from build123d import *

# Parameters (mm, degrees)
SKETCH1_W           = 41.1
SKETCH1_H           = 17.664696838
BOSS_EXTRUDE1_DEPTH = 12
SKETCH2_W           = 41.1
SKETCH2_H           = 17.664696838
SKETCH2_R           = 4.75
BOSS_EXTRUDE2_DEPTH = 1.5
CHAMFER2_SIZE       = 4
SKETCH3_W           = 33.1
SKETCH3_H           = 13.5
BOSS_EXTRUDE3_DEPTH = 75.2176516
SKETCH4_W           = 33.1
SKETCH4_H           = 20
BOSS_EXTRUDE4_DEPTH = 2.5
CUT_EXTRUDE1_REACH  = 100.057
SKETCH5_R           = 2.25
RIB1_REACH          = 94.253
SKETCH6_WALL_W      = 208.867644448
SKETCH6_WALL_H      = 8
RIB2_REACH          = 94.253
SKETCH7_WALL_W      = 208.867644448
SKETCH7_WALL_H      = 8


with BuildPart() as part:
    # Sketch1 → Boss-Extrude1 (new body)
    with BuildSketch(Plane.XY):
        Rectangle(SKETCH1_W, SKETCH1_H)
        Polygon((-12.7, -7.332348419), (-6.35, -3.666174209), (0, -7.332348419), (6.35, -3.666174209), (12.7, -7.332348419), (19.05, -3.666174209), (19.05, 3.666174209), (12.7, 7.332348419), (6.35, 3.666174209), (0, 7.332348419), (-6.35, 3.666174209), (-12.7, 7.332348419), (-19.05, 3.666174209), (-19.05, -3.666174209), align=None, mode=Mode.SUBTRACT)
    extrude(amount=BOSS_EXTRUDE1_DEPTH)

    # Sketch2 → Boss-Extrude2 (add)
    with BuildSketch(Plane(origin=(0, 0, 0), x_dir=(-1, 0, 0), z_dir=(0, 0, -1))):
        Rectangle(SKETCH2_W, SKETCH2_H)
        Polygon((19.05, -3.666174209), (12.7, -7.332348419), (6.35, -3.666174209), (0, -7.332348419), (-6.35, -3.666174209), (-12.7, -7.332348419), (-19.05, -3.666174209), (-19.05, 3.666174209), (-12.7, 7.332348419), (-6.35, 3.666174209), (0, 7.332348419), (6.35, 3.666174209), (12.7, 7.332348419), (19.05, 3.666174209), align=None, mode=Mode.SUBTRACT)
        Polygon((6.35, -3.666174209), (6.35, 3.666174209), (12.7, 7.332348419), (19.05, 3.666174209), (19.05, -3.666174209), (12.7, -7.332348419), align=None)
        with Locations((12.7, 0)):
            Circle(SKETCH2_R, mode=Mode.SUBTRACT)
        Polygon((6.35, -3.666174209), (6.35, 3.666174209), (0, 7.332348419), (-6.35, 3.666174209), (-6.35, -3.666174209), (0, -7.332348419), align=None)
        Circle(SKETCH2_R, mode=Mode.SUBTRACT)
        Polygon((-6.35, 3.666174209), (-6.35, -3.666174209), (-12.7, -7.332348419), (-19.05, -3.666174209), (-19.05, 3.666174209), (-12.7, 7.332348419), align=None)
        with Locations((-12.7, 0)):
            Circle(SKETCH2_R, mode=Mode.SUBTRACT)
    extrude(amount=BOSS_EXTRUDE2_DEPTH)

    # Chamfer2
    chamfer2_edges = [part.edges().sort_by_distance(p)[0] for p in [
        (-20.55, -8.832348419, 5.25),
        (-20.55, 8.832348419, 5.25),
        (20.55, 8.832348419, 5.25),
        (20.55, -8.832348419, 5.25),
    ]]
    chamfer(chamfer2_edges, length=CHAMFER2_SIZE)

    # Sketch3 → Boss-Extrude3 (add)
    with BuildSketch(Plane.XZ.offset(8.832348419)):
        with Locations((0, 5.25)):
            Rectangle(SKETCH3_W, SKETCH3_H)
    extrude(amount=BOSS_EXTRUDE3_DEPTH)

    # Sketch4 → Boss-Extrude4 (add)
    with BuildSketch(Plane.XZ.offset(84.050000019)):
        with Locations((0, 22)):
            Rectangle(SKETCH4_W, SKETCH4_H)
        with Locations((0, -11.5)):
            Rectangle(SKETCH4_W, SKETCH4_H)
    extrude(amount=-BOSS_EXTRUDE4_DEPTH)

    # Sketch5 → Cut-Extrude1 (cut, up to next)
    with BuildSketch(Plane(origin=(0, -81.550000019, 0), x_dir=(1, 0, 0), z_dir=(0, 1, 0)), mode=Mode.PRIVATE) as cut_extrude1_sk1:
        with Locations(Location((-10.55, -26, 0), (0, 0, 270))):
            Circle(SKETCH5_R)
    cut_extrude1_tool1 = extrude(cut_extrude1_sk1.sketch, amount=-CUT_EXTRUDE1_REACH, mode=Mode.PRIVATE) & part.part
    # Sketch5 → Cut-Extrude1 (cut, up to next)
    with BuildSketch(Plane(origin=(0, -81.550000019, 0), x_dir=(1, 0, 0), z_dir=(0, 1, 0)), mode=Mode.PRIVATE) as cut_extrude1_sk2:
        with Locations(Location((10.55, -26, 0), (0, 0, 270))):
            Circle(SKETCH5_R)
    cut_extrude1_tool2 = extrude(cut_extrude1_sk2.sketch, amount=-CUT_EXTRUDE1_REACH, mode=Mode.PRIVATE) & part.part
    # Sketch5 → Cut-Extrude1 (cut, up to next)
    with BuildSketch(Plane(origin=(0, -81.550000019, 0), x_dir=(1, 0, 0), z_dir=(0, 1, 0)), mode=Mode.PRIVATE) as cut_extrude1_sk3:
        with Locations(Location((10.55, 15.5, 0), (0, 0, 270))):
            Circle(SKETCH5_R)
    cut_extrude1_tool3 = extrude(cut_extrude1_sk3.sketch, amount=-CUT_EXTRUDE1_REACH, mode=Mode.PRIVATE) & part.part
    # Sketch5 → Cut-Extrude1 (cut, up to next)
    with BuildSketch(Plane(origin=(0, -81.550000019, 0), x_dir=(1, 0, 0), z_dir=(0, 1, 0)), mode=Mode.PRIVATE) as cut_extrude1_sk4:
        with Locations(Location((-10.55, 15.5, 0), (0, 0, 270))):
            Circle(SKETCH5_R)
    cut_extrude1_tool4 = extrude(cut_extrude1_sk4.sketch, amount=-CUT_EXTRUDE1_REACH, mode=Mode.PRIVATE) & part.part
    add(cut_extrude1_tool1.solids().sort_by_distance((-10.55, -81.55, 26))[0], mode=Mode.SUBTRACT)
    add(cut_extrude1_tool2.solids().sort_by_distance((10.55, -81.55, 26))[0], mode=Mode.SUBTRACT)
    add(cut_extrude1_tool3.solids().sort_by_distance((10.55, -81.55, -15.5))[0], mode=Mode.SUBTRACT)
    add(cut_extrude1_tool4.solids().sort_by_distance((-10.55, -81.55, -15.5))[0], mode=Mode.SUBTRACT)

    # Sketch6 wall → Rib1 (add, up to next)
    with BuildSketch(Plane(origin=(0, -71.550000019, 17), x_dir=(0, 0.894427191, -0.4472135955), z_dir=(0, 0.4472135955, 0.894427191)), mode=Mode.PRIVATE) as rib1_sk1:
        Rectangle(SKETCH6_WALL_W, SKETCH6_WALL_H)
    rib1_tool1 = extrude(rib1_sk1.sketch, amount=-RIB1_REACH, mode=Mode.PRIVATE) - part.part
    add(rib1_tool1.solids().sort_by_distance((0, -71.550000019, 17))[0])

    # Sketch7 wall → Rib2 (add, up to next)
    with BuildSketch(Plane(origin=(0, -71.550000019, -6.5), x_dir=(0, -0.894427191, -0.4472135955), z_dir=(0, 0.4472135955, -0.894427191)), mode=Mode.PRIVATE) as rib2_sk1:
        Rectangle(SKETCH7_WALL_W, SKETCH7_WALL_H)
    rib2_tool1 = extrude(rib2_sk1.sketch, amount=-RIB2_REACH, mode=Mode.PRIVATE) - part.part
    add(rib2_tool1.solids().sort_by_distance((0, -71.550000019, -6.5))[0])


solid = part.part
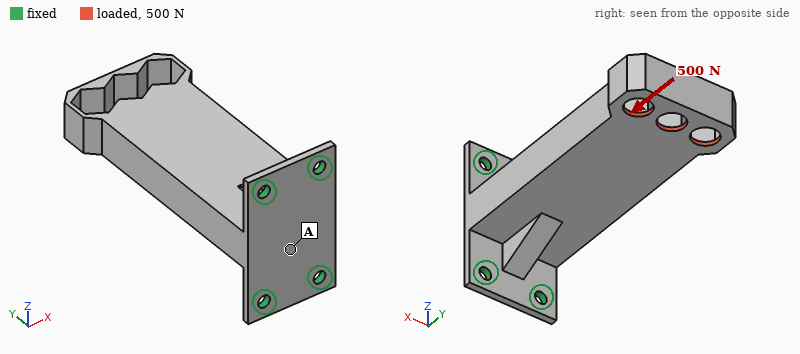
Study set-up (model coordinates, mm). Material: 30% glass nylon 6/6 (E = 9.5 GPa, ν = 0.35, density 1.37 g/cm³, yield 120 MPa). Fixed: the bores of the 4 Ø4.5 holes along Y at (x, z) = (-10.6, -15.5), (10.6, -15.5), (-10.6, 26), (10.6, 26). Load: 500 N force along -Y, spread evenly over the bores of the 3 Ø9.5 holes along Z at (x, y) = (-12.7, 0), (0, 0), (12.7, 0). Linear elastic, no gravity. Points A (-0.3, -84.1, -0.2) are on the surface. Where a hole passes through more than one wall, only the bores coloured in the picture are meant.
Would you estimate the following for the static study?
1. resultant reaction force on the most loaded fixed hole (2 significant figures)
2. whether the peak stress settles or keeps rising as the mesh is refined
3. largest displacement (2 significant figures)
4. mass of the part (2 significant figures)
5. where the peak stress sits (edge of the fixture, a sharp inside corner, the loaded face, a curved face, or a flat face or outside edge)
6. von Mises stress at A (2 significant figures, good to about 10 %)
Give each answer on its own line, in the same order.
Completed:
190 N
keeps rising
0.30 mm
58 g
edge of the fixture
4.8 MPa
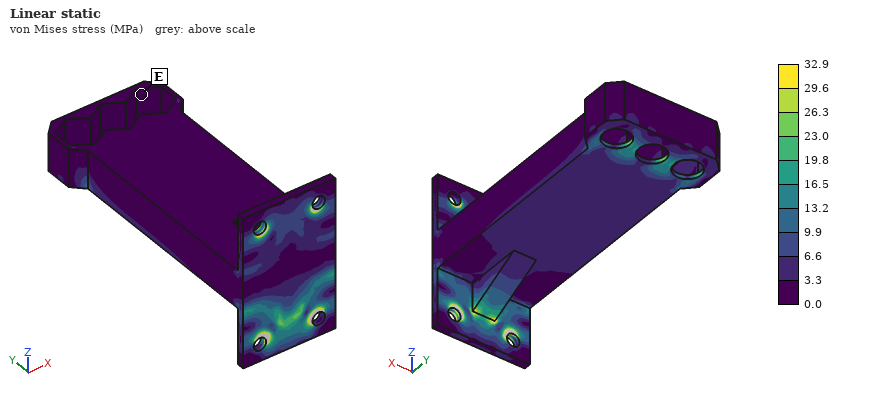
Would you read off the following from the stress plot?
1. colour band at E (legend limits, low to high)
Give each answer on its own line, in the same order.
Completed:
0.0 to 3.3 MPa
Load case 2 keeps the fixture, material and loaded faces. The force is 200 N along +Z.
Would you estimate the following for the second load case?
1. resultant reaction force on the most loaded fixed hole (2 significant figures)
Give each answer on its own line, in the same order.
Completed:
250 N
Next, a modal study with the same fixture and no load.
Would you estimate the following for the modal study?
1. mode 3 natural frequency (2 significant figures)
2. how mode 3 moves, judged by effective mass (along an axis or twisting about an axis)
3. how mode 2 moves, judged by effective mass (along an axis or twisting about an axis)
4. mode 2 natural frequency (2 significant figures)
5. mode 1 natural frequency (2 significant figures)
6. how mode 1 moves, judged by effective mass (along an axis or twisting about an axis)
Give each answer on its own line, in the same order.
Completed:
1900 Hz
along Y
along Z
590 Hz
330 Hz
along X
